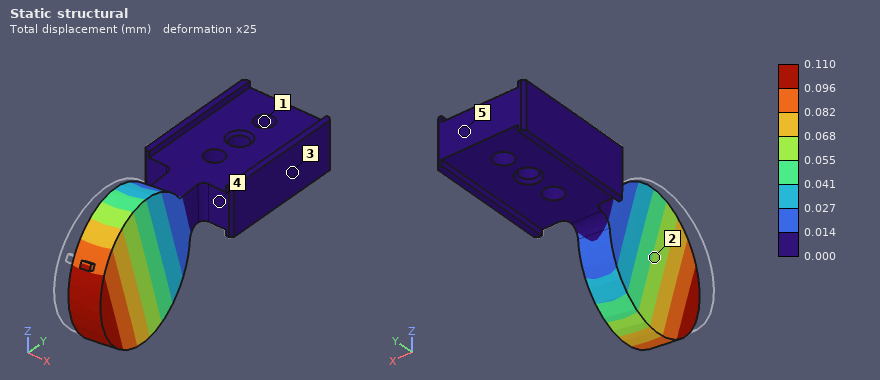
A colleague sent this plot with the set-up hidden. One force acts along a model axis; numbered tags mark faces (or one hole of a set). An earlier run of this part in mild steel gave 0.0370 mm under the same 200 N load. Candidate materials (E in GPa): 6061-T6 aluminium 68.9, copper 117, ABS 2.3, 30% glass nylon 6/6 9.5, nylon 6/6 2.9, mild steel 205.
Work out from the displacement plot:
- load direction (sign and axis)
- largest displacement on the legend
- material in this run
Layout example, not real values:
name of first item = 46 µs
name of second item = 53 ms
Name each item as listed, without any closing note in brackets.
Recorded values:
load direction = +X
largest displacement on the legend = 0.110 mm
material in this run = 6061-T6 aluminium
